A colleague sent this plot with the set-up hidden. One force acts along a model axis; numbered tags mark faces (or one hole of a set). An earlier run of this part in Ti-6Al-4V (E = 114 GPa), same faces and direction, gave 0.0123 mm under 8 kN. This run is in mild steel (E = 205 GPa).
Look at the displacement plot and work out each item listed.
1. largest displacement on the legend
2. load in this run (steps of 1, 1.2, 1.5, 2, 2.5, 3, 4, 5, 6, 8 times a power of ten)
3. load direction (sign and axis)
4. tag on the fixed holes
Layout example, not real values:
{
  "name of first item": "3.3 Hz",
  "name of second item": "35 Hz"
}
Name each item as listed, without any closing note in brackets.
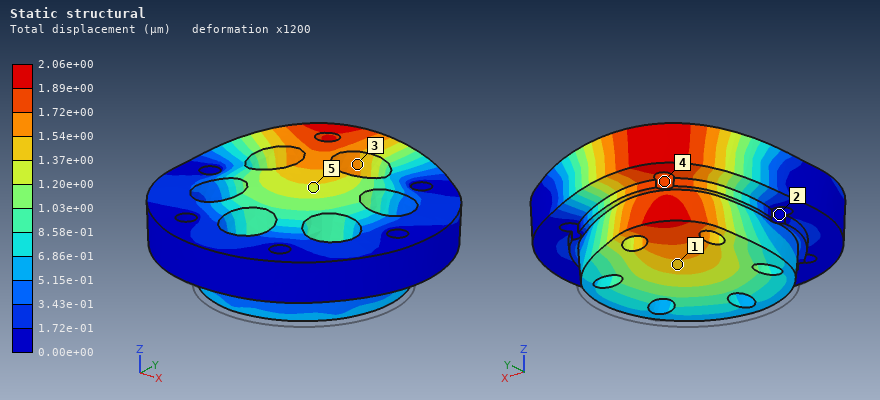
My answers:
{
  "largest displacement on the legend": "2.06e+00 µm",
  "load in this run": "2.5 kN",
  "load direction": "+Z",
  "tag on the fixed holes": "2"
}
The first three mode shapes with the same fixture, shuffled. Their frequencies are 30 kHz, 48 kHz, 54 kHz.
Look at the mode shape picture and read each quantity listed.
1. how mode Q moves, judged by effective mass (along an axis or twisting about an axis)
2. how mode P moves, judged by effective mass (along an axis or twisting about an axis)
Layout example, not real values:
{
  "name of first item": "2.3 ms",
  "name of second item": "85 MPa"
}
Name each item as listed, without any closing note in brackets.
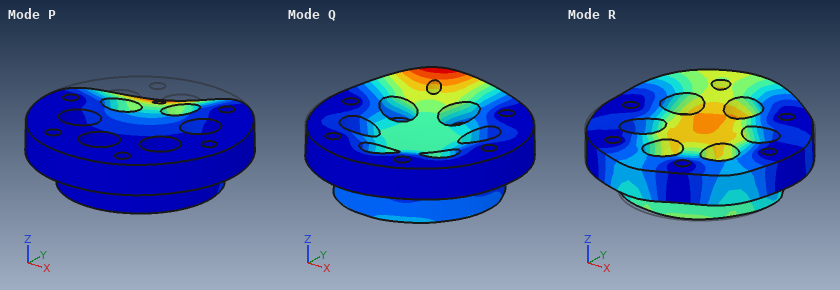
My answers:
{
  "how mode Q moves, judged by effective mass": "along Z",
  "how mode P moves, judged by effective mass": "along Z"
}
